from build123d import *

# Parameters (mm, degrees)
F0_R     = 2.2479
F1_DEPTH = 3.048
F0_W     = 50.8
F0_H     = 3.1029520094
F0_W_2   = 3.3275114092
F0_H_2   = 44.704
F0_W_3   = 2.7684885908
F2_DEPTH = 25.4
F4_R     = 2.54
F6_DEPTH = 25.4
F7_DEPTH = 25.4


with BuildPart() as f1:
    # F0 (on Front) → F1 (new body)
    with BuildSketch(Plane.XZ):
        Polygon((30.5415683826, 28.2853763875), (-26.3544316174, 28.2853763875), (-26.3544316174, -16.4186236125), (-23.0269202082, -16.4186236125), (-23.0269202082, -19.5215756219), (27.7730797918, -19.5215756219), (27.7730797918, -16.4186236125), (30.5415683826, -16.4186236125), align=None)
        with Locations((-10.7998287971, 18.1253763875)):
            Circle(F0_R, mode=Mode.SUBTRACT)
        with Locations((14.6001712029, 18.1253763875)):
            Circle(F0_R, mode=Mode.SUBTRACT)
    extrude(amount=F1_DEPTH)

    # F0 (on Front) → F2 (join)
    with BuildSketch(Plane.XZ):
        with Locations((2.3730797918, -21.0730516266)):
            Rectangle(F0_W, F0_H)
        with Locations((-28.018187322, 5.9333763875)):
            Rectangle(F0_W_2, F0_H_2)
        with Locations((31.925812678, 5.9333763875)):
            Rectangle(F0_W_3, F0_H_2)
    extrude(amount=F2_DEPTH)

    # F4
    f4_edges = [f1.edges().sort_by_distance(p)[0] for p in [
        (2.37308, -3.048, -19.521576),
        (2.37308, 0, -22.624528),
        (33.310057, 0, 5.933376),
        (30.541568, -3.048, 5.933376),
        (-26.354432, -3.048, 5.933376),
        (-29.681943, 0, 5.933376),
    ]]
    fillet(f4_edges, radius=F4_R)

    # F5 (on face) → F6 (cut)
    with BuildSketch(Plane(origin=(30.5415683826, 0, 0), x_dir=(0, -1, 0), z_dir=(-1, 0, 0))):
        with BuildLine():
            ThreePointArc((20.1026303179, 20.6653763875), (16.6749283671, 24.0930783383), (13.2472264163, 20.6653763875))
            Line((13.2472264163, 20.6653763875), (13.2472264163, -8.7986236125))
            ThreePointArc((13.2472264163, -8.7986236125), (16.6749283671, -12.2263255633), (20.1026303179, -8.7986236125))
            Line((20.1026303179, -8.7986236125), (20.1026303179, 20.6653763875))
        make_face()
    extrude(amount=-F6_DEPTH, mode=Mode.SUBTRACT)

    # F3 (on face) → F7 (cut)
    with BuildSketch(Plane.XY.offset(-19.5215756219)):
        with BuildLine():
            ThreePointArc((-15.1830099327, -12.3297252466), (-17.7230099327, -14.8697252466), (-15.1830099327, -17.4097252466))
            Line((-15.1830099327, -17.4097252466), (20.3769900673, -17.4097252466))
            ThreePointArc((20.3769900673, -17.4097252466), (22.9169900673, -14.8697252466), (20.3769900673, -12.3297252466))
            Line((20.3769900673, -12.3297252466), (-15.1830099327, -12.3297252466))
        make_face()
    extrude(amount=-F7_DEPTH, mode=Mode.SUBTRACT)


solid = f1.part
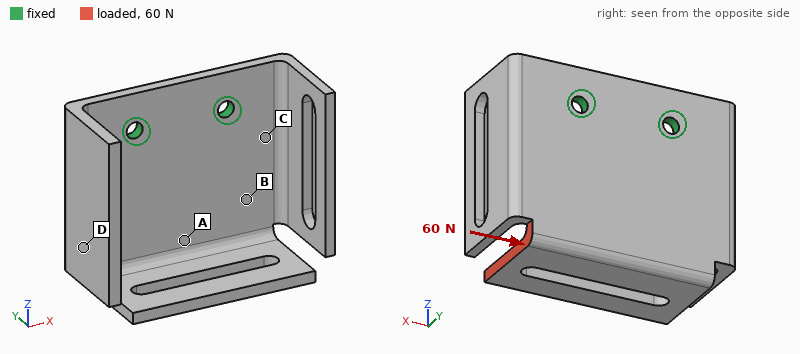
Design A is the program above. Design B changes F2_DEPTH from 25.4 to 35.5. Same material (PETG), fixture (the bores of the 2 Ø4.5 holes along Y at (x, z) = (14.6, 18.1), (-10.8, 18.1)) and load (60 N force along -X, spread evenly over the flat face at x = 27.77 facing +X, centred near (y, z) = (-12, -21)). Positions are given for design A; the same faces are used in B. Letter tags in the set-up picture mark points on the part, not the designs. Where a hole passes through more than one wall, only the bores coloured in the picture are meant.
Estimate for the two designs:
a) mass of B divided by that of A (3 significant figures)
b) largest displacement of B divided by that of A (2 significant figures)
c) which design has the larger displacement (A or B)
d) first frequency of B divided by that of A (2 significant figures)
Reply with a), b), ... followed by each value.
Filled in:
a) 1.24
b) 1.8
c) B
d) 0.74
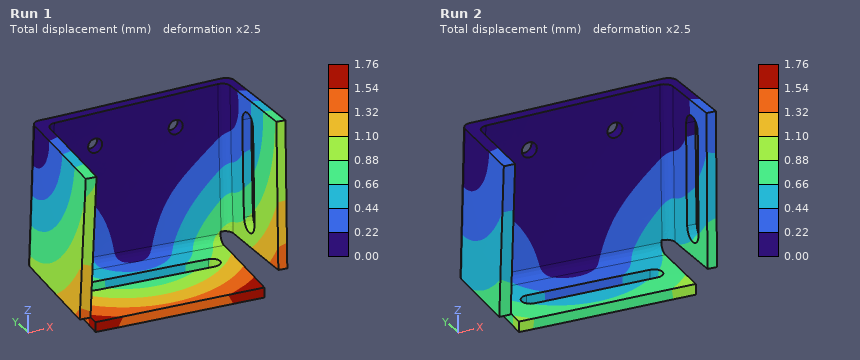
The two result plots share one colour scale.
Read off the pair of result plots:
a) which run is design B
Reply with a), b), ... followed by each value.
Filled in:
a) Run 1
